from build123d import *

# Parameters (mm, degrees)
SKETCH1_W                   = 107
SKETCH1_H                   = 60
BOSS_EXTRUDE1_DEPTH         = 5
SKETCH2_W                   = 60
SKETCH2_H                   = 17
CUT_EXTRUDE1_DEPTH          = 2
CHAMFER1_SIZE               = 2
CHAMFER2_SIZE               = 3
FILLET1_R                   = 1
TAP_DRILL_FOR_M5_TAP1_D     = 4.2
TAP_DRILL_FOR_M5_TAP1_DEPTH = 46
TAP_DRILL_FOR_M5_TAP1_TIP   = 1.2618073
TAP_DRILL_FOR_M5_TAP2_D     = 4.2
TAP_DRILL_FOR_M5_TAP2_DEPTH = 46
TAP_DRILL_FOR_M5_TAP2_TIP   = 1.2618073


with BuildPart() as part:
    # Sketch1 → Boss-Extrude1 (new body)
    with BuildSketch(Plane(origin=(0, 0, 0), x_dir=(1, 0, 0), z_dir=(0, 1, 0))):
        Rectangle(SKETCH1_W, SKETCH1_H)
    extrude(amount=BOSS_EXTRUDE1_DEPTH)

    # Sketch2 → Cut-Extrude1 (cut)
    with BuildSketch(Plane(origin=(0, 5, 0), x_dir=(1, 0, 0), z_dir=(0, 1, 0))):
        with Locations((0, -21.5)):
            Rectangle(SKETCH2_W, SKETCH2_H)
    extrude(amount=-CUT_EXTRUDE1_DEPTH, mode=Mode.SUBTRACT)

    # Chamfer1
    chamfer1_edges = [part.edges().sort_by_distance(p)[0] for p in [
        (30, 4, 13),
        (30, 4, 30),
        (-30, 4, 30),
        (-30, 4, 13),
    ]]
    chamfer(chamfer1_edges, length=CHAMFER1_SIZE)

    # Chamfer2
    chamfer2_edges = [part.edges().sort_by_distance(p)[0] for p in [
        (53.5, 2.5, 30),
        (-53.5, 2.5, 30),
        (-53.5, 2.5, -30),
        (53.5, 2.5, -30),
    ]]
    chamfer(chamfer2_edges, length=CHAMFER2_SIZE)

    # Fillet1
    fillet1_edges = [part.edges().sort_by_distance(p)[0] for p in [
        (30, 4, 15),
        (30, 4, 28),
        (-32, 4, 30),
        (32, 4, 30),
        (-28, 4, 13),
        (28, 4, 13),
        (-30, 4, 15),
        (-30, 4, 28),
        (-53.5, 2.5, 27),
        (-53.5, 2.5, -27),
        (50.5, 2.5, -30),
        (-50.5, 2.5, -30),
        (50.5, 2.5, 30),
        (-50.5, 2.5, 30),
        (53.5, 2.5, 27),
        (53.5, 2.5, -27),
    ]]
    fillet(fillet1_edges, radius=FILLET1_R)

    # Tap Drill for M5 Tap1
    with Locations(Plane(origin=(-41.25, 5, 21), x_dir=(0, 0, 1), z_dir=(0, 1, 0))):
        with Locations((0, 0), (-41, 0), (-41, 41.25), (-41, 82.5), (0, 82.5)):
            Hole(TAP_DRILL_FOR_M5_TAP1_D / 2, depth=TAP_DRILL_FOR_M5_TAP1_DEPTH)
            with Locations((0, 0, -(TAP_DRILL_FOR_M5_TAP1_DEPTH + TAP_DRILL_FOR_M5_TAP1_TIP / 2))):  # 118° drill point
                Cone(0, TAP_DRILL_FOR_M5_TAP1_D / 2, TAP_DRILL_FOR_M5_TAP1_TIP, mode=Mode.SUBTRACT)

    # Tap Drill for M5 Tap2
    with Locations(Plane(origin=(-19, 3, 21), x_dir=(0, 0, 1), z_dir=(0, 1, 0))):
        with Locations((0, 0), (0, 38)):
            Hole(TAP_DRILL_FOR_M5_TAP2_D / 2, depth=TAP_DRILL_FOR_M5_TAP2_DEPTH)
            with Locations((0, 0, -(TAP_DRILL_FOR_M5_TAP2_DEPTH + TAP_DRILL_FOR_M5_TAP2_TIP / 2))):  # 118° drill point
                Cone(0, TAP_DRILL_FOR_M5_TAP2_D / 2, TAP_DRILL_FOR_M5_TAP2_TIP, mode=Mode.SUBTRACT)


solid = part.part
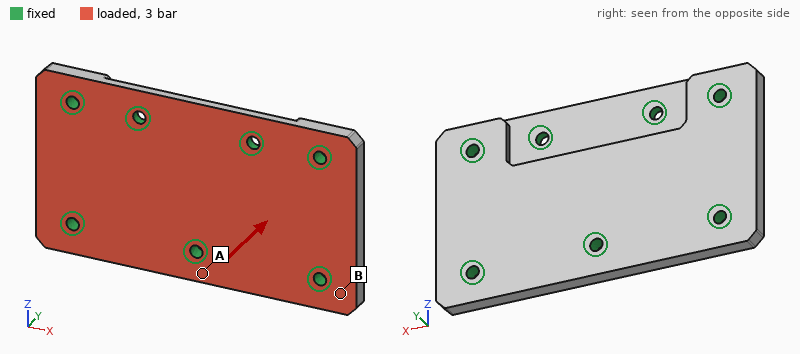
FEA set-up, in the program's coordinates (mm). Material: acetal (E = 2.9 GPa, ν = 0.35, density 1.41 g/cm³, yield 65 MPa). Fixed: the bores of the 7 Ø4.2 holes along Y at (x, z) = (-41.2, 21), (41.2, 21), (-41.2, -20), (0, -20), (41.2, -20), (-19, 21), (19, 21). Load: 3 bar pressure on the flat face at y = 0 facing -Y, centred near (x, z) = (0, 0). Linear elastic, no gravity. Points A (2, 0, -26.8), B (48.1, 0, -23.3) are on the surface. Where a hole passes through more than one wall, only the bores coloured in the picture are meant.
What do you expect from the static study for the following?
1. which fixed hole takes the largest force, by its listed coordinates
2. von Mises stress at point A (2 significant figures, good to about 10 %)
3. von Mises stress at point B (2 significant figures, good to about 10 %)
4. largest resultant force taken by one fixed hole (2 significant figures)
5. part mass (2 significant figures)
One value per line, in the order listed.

(0, -20)
5.8 MPa
2.6 MPa
400 N
42 g
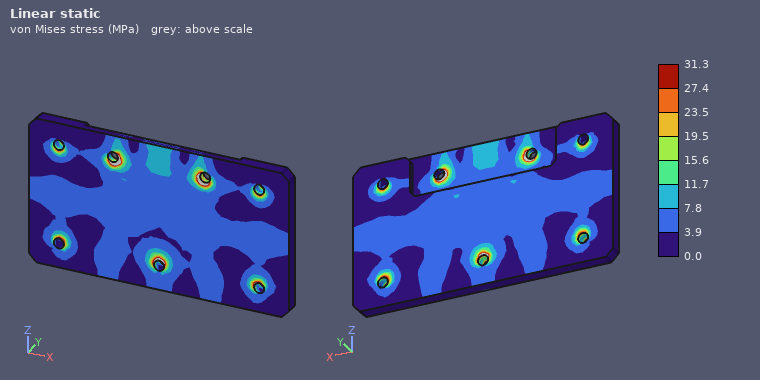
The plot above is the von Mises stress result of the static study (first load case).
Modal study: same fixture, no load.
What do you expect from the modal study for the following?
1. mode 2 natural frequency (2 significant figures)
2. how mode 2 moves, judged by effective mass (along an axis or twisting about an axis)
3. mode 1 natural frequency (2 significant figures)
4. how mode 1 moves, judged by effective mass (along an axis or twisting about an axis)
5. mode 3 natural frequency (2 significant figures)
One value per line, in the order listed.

3300 Hz
twisting about Z
2800 Hz
along Y
3500 Hz
